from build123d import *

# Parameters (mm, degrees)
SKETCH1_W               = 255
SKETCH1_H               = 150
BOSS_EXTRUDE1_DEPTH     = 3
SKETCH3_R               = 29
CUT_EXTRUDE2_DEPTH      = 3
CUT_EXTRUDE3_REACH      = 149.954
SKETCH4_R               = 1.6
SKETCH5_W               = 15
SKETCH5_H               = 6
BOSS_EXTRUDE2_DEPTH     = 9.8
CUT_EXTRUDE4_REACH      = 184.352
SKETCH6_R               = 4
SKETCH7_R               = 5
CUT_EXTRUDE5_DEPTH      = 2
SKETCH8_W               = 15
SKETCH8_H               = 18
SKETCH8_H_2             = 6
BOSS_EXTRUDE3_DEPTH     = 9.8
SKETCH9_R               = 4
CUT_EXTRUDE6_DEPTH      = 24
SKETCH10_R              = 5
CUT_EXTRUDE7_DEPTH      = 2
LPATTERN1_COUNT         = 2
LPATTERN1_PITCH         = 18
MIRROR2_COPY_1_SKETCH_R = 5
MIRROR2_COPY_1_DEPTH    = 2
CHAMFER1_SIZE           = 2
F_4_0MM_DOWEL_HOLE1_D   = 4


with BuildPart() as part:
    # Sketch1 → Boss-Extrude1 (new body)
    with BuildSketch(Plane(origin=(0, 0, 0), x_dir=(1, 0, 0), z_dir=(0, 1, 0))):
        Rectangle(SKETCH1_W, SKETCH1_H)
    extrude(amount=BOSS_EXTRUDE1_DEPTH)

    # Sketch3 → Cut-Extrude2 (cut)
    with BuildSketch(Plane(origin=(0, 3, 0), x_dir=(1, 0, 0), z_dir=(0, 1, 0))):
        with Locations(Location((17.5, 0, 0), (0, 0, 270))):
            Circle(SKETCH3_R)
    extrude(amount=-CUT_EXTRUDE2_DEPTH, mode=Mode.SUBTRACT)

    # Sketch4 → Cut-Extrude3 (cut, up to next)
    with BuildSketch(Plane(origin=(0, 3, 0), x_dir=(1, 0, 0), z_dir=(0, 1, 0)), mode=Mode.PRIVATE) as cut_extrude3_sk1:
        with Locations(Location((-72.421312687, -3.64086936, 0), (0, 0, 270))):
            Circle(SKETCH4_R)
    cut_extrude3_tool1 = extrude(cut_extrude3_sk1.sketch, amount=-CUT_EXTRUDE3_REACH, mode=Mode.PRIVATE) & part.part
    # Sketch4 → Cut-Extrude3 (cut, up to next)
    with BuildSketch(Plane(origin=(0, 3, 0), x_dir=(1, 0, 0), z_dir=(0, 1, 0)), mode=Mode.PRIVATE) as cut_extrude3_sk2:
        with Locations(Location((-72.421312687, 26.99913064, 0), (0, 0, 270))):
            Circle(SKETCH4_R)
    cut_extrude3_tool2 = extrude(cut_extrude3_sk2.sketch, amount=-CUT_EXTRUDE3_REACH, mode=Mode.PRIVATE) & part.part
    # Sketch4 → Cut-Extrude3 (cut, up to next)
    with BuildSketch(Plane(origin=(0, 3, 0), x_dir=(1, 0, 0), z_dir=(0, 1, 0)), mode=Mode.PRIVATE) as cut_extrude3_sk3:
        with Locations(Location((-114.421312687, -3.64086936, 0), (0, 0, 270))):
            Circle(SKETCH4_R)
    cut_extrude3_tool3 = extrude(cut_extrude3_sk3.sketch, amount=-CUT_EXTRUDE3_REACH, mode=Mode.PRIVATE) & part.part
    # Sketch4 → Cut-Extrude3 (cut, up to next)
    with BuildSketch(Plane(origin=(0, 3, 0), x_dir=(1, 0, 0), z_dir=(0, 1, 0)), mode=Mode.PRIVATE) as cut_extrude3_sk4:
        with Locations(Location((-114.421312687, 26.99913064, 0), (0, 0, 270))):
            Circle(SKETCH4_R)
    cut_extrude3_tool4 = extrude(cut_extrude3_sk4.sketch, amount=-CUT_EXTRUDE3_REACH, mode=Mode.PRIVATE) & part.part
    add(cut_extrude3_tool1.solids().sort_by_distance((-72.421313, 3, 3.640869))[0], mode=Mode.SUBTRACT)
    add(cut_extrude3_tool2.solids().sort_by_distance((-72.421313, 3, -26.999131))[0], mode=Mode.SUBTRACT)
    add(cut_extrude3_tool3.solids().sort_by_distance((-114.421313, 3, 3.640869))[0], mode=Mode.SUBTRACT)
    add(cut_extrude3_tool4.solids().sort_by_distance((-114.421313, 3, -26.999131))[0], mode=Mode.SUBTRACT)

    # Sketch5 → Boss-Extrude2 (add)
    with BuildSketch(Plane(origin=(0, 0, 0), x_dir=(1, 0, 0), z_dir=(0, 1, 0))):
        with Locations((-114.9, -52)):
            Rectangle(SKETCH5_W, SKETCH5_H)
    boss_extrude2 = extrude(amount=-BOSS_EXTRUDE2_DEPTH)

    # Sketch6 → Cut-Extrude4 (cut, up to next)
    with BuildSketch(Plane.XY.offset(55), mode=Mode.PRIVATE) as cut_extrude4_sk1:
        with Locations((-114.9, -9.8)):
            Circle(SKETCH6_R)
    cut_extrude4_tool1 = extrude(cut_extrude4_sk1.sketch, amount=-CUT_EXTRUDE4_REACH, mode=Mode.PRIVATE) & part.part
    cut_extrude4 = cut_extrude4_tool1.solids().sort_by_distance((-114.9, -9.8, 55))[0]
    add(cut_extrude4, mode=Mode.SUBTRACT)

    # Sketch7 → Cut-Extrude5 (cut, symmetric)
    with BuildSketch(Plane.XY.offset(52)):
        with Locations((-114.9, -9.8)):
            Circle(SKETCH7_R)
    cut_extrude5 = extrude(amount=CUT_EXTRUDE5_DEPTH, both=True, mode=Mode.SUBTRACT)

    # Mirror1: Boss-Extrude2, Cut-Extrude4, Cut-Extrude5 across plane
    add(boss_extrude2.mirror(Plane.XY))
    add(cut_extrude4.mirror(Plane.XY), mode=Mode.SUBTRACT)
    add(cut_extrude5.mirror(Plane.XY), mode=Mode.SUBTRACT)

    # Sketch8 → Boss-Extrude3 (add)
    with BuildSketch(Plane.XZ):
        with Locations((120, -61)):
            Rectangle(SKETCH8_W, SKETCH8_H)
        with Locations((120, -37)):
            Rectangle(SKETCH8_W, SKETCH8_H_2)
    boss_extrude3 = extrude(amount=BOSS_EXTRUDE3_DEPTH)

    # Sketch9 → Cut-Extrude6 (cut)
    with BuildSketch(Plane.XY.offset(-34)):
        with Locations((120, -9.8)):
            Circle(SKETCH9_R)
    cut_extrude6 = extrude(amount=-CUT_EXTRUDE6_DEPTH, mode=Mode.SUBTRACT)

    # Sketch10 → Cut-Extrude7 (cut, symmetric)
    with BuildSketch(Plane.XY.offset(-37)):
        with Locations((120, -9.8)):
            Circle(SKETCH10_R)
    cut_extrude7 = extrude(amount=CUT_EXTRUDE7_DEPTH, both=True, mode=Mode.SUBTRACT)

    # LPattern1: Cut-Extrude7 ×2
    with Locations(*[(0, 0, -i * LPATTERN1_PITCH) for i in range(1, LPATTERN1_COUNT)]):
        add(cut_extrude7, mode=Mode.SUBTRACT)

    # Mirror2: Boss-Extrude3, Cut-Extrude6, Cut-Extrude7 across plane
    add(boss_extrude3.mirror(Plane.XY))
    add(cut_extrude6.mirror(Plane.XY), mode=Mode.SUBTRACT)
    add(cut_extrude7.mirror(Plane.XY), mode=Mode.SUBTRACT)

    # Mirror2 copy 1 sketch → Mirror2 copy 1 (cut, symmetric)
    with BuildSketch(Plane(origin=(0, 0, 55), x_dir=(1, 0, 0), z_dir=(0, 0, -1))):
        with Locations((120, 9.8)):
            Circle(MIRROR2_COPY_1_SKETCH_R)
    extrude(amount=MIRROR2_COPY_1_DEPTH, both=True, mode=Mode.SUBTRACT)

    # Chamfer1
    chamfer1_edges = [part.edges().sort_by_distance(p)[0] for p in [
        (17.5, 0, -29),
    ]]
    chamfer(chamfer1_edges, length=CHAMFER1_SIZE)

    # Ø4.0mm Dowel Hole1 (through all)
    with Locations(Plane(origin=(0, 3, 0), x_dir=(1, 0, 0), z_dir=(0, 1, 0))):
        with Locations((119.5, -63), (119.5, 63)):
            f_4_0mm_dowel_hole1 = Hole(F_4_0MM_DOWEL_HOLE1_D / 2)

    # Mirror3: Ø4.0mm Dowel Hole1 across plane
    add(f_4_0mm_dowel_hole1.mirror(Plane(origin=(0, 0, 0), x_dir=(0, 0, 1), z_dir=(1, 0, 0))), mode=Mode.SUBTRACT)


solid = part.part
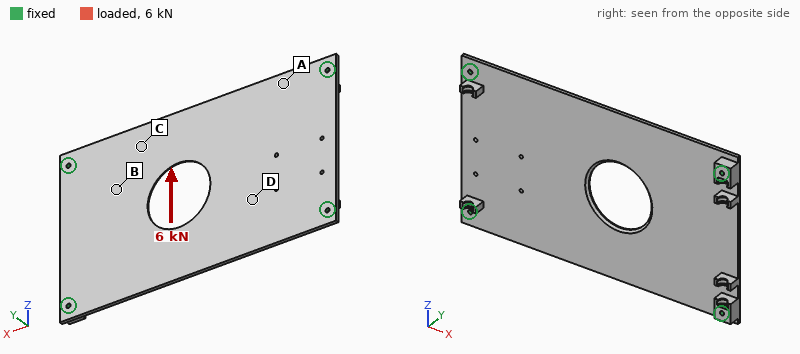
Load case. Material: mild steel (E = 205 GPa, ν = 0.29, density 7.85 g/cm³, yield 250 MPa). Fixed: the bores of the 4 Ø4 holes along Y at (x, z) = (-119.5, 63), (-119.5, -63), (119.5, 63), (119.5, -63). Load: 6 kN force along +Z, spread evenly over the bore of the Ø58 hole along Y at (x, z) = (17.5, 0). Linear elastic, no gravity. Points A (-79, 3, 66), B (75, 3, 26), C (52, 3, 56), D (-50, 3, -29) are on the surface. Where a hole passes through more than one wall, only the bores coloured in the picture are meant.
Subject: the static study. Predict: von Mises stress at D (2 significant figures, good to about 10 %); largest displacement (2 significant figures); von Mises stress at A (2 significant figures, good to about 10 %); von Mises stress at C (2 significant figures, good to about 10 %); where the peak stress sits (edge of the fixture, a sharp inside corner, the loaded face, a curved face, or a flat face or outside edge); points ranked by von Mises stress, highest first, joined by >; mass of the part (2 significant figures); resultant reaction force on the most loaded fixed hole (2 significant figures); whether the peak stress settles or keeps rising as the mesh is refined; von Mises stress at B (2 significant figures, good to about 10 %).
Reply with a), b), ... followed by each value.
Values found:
a) 18 MPa
b) 90 µm
c) 8.6 MPa
d) 14 MPa
e) edge of the fixture
f) B > D > C > A
g) 890 g
h) 2.1 kN
i) keeps rising
j) 25 MPa
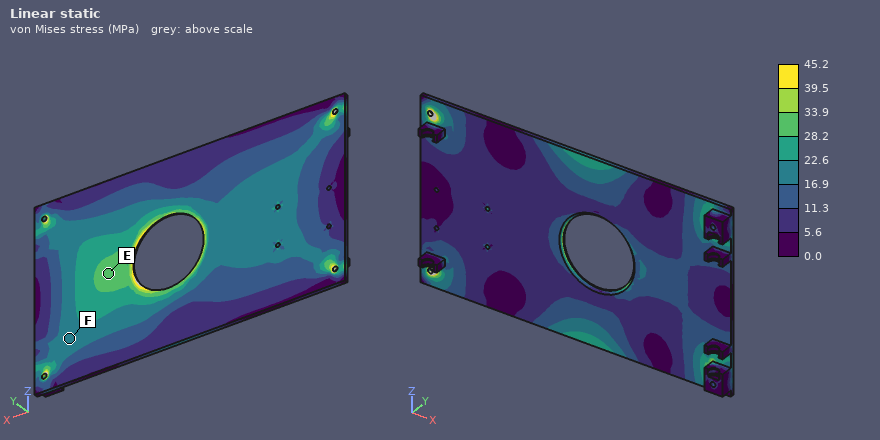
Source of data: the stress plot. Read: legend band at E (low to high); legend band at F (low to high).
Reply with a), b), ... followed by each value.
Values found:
a) 28.2 to 33.9 MPa
b) 16.9 to 22.6 MPa
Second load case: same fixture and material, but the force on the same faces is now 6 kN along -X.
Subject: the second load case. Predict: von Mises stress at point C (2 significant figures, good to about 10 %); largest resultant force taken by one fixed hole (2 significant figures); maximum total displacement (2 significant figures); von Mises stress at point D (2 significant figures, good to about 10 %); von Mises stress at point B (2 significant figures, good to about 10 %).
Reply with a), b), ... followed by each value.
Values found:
a) 10 MPa
b) 1.8 kN
c) 50 µm
d) 10 MPa
e) 12 MPa
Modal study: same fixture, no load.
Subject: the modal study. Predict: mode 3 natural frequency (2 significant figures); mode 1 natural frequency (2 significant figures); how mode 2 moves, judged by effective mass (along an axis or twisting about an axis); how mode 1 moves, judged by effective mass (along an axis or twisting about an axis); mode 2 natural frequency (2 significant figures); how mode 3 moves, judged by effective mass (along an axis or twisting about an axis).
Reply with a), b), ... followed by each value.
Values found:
a) 650 Hz
b) 250 Hz
c) twisting about X
d) along Y
e) 410 Hz
f) twisting about Z
